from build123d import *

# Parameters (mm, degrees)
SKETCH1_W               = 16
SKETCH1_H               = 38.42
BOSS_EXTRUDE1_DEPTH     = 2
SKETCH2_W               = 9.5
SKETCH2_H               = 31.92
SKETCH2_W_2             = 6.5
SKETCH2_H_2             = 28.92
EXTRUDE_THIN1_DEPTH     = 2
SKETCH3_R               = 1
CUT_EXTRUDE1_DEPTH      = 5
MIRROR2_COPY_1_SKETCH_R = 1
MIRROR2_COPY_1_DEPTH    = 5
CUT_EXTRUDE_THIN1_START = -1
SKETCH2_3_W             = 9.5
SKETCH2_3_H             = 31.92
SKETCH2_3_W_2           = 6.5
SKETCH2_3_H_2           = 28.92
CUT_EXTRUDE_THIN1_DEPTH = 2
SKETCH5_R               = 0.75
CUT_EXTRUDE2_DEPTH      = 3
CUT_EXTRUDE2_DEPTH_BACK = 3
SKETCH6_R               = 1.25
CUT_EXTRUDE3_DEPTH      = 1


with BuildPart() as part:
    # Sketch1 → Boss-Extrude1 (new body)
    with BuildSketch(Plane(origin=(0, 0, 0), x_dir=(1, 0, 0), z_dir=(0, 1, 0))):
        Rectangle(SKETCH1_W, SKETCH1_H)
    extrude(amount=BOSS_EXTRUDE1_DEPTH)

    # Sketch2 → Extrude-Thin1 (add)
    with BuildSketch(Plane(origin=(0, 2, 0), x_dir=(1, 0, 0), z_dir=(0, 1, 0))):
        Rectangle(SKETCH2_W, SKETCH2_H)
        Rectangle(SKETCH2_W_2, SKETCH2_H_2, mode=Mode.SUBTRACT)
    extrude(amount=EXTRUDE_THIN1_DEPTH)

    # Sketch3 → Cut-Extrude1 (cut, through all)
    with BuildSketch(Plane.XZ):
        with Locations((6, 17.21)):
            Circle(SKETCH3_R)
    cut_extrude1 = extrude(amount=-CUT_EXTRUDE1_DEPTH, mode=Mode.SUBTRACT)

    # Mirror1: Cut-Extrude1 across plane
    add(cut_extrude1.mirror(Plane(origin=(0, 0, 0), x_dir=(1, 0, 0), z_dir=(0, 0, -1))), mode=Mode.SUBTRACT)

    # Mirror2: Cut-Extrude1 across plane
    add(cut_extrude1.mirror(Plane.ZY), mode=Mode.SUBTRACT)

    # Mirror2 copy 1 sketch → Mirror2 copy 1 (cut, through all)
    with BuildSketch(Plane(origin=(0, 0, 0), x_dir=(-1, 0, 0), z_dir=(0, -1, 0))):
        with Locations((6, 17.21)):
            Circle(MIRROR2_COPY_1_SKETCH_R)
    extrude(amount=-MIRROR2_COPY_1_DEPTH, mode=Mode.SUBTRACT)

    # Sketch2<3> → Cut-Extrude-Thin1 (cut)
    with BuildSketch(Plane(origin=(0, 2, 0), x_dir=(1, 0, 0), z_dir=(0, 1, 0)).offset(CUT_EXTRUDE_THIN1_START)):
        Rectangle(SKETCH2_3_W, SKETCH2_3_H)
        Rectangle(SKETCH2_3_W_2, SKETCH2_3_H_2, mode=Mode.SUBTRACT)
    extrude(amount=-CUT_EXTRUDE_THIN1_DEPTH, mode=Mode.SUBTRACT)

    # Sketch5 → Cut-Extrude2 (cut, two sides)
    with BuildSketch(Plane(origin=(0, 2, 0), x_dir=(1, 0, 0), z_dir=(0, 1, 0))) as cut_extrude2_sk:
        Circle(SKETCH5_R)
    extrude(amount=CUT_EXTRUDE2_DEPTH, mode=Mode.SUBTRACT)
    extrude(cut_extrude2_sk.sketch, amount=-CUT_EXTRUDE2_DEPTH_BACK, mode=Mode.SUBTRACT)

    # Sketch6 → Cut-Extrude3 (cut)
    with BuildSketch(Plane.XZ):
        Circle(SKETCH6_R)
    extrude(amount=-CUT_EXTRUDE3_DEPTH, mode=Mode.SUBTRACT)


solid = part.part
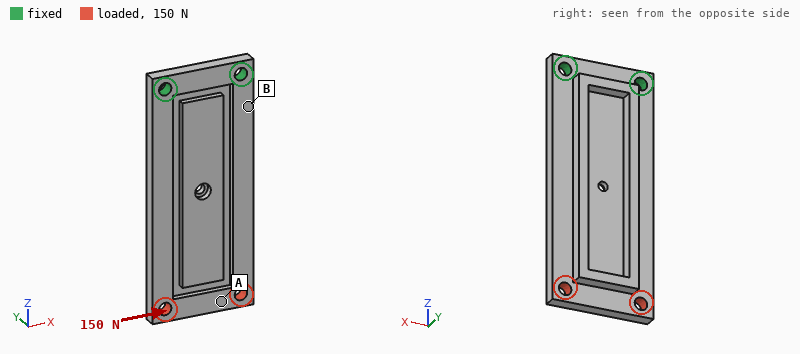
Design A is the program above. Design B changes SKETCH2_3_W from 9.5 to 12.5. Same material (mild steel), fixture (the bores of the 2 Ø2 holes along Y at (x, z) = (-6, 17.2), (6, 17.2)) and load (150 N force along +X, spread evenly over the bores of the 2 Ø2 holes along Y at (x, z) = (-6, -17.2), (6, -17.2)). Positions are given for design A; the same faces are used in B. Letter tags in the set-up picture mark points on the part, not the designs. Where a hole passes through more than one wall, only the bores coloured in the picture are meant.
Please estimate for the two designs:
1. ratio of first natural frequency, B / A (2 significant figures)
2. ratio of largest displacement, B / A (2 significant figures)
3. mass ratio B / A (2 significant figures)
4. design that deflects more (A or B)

0.90
1.2
0.93
B
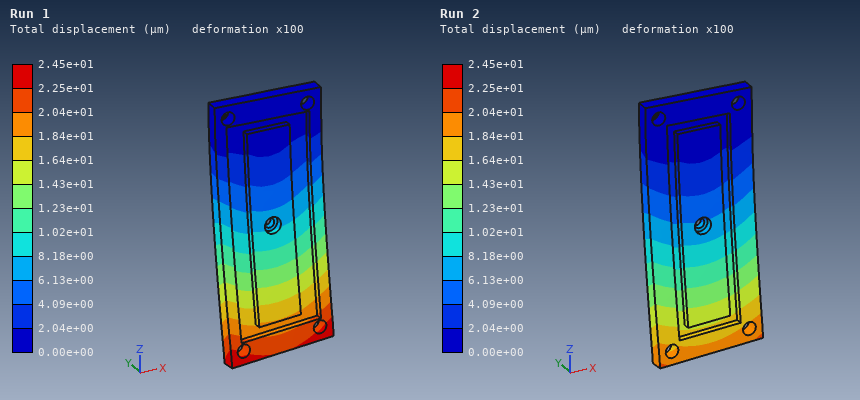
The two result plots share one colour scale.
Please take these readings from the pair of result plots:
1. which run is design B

Run 1
